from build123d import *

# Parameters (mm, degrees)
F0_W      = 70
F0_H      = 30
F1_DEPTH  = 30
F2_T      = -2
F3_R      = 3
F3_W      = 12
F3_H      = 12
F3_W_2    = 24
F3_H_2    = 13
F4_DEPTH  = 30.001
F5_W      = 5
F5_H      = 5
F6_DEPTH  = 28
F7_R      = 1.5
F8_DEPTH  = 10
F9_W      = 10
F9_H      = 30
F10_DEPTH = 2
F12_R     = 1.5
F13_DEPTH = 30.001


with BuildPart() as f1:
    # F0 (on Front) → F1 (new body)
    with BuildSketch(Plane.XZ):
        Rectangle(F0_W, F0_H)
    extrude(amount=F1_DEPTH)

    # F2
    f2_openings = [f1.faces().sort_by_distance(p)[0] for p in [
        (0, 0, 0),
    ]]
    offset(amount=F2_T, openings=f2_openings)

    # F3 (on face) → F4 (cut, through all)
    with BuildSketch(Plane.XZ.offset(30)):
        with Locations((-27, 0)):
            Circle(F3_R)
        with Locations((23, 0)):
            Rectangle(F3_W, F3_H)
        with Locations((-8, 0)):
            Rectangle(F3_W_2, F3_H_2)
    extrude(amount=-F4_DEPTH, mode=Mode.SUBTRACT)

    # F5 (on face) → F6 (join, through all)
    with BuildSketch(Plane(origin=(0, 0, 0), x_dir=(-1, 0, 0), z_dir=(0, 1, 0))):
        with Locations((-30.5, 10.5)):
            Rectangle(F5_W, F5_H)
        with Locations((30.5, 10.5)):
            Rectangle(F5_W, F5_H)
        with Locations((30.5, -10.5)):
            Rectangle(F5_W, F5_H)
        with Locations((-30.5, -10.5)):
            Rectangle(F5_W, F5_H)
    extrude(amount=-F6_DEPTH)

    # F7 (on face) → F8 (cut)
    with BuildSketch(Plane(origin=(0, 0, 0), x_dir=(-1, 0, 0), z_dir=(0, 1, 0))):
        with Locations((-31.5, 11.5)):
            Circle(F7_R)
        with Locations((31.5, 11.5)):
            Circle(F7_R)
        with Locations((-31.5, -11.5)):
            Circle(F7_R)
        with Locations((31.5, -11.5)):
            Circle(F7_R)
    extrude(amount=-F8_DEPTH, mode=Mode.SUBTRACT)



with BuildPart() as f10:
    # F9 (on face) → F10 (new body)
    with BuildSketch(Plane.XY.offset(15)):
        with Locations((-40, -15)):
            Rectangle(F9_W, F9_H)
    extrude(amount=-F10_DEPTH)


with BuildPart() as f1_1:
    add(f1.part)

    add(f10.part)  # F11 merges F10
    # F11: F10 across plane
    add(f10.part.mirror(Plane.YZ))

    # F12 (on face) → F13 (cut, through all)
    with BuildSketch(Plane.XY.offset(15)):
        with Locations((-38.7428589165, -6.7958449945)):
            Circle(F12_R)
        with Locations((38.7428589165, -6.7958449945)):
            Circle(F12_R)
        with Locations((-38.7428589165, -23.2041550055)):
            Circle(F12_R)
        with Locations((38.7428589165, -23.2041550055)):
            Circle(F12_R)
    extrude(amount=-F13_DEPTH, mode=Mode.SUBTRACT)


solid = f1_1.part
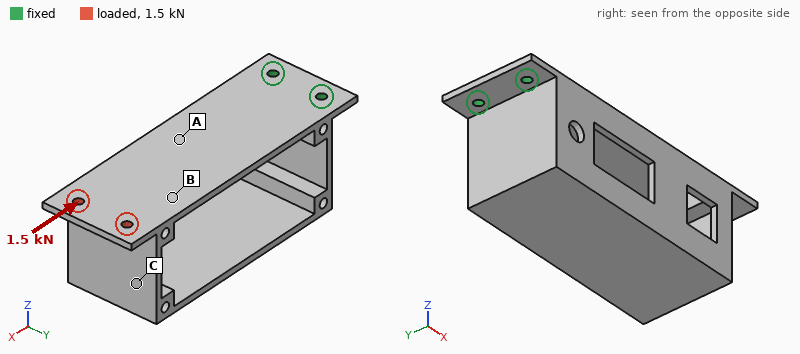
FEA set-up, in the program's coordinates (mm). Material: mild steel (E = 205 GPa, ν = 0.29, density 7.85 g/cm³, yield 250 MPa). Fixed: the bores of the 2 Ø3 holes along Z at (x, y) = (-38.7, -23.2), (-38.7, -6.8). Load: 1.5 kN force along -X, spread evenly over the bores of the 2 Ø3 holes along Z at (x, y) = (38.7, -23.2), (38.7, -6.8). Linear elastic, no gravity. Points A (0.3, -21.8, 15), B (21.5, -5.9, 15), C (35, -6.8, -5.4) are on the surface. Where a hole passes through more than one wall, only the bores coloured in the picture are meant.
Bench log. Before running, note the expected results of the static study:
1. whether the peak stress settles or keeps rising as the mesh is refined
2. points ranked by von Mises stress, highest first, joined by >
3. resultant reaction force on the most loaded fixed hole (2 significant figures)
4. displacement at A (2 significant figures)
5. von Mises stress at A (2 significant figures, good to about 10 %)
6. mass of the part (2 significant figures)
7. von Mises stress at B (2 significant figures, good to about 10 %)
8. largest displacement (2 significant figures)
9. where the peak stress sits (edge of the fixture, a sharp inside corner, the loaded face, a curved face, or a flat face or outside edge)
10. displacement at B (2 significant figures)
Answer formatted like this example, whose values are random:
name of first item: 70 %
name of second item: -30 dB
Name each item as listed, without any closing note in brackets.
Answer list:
whether the peak stress settles or keeps rising as the mesh is refined: keeps rising
points ranked by von Mises stress, highest first, joined by >: B > A > C
resultant reaction force on the most loaded fixed hole: 750 N
displacement at A: 8.6 µm
von Mises stress at A: 20 MPa
mass of the part: 140 g
von Mises stress at B: 27 MPa
largest displacement: 27 µm
where the peak stress sits: edge of the fixture
displacement at B: 16 µm
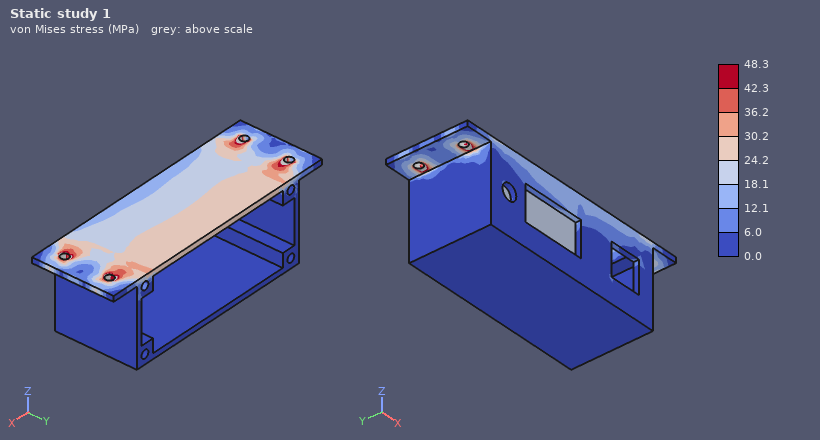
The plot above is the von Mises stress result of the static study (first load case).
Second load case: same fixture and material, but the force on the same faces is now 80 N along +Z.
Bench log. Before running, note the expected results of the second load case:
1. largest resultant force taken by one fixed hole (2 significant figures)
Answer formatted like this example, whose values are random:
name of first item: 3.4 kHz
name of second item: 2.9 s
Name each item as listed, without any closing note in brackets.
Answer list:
largest resultant force taken by one fixed hole: 42 N
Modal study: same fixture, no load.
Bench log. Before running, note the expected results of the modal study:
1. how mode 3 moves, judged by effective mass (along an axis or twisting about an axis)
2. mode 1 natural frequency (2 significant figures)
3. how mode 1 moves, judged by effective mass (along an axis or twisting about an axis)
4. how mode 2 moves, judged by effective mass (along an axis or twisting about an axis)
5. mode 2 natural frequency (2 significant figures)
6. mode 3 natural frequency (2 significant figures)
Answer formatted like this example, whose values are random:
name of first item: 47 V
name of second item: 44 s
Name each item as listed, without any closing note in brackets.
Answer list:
how mode 3 moves, judged by effective mass: along Y
mode 1 natural frequency: 240 Hz
how mode 1 moves, judged by effective mass: along Z
how mode 2 moves, judged by effective mass: along Y
mode 2 natural frequency: 960 Hz
mode 3 natural frequency: 2300 Hz
